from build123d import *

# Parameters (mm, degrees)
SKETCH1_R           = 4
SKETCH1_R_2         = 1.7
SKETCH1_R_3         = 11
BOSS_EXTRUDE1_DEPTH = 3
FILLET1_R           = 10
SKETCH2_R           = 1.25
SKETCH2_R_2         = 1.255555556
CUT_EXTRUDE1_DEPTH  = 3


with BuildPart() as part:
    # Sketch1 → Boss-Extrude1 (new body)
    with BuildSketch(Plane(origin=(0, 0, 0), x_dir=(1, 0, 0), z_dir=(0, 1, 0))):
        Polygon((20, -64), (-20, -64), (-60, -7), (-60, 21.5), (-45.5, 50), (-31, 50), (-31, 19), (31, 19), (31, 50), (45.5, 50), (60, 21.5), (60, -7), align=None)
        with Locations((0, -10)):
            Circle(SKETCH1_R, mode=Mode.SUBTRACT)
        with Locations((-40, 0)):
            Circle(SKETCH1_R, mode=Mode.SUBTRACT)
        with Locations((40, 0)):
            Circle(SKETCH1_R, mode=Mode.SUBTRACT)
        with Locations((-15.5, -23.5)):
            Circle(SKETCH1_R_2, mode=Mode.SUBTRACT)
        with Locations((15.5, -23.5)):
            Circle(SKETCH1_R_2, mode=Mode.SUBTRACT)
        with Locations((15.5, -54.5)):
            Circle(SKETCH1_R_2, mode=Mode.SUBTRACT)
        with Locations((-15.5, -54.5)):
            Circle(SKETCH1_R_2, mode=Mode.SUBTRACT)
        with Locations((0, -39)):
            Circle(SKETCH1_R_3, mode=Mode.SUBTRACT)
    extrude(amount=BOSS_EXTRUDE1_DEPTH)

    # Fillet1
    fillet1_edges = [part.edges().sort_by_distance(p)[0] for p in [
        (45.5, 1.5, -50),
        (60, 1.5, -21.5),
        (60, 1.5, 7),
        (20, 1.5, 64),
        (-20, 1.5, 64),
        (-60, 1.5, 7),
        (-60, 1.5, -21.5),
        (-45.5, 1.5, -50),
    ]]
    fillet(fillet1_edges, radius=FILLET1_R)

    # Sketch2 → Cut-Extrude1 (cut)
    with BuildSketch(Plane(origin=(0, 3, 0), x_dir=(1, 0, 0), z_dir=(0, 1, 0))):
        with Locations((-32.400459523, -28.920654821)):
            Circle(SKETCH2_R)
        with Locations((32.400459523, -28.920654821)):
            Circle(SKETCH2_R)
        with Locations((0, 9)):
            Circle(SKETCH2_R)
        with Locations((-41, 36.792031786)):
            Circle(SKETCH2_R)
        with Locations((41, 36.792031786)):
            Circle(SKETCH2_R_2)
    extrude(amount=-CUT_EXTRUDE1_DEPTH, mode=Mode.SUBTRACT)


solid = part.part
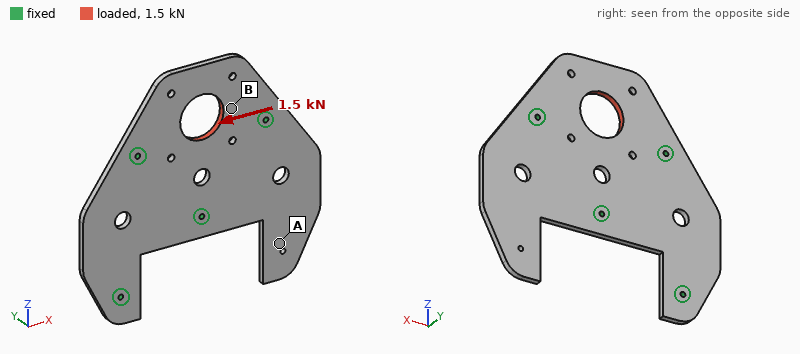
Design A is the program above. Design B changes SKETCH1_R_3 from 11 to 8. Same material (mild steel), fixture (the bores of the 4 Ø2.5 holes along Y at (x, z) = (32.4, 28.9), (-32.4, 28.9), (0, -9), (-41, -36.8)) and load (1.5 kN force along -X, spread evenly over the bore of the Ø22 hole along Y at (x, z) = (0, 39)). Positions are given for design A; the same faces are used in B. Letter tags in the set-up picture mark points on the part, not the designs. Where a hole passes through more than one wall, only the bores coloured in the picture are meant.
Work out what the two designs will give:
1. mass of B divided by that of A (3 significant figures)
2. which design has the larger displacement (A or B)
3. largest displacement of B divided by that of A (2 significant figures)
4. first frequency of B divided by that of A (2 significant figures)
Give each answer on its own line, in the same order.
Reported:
1.02
A
0.87
1.0
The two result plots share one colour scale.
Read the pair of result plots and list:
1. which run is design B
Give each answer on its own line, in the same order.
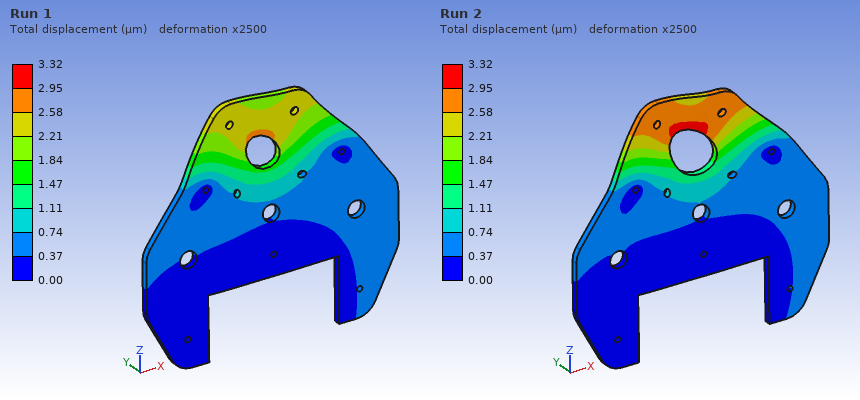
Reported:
Run 1
